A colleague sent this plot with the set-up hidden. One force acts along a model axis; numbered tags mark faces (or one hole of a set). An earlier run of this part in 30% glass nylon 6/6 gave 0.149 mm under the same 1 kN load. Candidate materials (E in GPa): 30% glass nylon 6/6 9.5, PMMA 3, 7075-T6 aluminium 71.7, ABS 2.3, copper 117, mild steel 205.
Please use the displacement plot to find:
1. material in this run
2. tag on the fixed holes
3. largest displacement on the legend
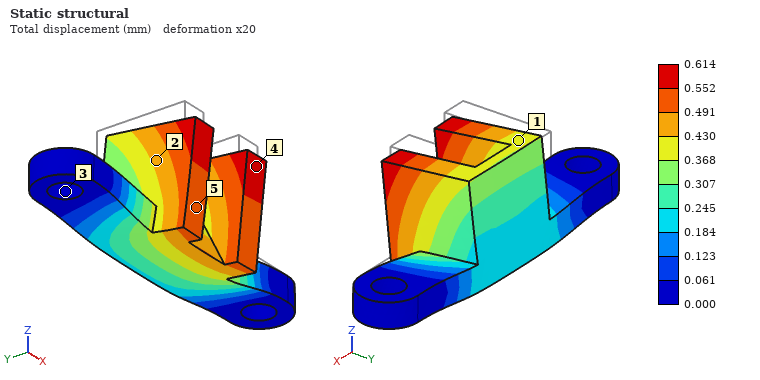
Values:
ABS
3
0.614 mm
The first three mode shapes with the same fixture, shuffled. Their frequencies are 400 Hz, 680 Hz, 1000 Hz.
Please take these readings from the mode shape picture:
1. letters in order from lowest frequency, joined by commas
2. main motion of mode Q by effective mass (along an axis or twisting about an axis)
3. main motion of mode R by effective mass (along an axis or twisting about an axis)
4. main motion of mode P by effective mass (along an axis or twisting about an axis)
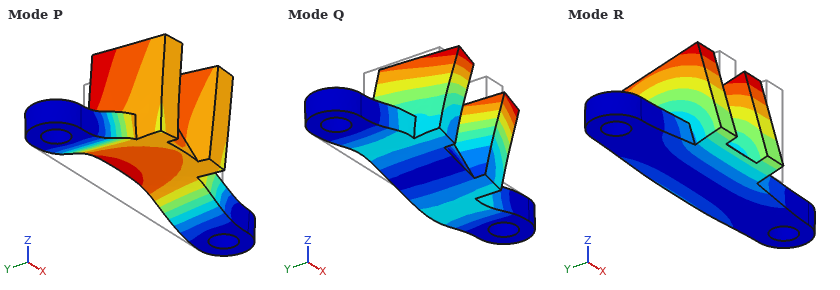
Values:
R, P, Q
along X
along Y
along Z
